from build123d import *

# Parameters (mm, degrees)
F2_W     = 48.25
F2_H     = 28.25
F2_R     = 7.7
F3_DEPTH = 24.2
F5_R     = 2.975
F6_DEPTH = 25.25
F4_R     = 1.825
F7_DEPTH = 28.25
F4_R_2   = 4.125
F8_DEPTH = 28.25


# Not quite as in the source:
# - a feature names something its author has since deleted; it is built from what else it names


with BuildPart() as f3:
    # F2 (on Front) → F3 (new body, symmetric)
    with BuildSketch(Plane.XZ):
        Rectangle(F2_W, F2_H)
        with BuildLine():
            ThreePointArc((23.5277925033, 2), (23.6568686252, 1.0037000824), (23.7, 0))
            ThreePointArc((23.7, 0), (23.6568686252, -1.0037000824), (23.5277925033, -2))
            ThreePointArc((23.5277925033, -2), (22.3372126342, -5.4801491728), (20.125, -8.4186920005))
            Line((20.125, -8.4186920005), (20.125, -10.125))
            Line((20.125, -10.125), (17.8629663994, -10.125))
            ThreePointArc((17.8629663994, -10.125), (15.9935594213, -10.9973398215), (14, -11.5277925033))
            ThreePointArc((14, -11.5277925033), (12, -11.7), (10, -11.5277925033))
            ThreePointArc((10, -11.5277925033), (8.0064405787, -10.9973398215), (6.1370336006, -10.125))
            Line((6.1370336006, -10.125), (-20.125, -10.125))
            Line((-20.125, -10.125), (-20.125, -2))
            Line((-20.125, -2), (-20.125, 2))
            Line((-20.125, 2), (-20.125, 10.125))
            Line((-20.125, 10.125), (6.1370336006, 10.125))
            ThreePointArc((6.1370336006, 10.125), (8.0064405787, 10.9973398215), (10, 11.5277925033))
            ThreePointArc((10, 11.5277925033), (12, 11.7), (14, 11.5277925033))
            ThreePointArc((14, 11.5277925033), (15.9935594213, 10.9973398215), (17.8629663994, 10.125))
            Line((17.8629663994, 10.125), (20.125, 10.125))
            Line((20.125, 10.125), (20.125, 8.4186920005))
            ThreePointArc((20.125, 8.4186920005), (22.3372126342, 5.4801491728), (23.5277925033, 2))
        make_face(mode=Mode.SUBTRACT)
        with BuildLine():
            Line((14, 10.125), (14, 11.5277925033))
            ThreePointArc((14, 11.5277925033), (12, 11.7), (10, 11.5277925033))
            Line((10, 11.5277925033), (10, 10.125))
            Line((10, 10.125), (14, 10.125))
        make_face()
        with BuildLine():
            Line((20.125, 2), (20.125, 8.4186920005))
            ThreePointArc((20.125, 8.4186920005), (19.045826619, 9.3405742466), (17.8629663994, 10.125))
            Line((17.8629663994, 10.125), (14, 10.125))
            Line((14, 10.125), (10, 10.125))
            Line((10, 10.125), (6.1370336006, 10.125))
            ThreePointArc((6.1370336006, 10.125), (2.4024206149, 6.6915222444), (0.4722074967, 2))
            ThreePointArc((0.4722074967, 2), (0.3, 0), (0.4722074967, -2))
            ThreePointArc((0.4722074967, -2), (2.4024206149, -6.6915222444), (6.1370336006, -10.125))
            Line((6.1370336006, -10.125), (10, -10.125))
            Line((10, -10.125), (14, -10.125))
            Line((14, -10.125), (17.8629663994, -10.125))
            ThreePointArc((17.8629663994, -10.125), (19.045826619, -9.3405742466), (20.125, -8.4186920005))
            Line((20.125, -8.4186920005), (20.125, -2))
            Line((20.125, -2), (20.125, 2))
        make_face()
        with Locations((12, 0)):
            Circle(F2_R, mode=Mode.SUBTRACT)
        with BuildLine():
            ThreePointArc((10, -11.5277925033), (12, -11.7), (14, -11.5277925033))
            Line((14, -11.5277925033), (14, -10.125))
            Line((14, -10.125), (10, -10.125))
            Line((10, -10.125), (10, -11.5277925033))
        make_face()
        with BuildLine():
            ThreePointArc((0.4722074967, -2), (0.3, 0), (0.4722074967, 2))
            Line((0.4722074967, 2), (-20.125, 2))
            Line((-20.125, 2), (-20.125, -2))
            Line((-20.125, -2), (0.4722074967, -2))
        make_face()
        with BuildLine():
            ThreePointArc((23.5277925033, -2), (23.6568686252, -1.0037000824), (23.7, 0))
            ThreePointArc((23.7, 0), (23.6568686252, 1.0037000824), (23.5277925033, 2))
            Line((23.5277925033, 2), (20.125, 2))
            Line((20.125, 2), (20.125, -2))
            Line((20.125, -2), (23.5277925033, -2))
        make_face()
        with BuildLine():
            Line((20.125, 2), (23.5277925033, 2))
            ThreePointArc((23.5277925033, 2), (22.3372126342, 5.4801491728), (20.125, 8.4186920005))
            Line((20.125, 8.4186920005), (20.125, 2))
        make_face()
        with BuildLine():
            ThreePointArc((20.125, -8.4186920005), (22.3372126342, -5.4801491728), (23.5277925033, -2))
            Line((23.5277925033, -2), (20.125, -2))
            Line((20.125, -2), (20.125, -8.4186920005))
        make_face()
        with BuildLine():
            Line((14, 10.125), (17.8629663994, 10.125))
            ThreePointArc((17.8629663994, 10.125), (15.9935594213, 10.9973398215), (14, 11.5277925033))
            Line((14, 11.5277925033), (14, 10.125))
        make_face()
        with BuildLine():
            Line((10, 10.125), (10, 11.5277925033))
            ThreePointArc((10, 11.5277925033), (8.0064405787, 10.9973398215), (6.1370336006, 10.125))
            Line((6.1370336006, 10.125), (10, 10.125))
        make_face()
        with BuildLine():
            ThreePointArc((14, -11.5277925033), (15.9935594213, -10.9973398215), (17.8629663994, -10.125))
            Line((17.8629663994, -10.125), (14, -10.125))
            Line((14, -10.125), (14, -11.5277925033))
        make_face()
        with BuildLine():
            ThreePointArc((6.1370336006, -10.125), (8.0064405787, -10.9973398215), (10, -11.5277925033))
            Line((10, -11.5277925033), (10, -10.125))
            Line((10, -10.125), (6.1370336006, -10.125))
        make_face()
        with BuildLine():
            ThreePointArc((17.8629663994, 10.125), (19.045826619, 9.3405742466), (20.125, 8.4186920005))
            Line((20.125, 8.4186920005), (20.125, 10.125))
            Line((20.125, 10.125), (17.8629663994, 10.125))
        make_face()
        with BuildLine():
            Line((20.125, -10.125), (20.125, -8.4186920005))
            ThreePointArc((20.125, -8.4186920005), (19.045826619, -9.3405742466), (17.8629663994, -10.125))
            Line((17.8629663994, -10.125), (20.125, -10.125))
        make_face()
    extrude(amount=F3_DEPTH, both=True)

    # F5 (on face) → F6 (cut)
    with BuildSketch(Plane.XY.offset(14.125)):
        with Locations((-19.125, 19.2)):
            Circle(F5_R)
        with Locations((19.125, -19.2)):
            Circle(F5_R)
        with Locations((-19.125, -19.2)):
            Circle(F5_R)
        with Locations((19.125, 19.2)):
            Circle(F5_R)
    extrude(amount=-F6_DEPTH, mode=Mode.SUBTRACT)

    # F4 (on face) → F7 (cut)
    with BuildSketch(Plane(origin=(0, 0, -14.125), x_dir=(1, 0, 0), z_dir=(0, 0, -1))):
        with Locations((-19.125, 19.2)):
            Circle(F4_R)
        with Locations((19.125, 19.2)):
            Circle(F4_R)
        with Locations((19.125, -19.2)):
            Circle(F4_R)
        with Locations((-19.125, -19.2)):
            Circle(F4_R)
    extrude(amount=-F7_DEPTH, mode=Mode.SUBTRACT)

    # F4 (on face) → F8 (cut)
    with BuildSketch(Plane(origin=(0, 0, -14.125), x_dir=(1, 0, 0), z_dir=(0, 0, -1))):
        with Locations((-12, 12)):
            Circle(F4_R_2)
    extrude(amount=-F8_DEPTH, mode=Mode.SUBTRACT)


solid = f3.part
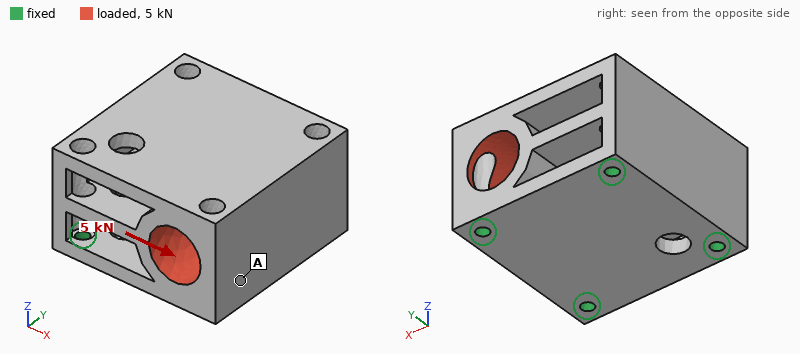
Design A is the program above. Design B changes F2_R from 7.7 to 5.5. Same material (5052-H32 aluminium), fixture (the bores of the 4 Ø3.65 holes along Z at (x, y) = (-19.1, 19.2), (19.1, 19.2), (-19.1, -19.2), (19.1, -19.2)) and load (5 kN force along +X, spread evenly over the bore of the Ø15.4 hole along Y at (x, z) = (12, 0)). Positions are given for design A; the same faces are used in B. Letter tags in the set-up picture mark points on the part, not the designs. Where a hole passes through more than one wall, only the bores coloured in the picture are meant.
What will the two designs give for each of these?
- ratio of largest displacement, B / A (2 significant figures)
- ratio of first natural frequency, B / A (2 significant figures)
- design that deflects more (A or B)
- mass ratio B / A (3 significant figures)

0.91
0.98
A
1.11
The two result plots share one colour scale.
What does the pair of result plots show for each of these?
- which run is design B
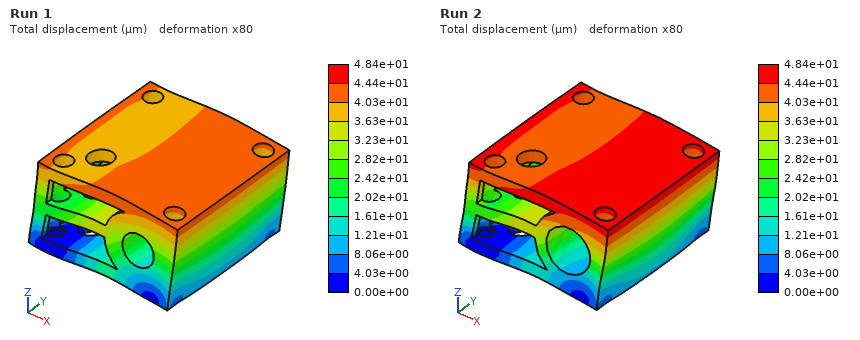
Run 1
